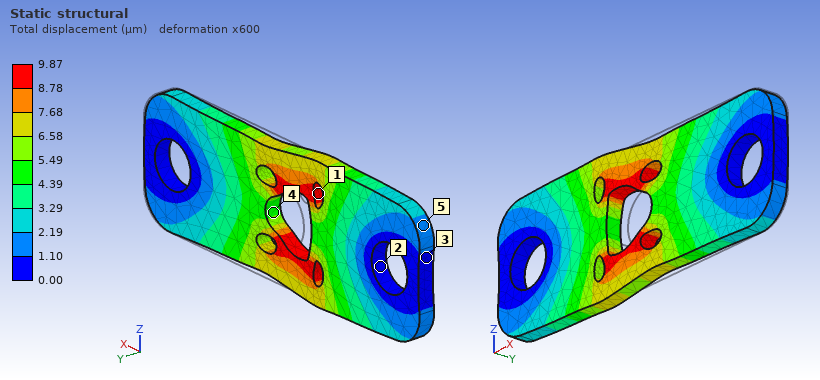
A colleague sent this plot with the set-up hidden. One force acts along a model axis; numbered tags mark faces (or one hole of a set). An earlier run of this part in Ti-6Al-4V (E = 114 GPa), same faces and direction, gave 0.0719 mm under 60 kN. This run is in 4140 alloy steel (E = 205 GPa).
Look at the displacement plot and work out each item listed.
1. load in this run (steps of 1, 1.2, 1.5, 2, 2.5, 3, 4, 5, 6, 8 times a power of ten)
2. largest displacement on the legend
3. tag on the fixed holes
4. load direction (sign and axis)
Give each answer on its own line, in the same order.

15 kN
9.87 µm
2
-X
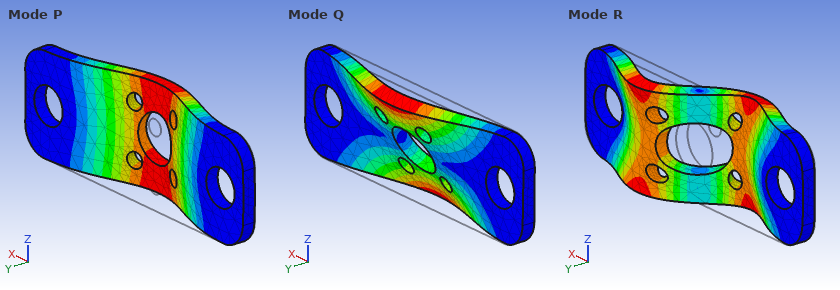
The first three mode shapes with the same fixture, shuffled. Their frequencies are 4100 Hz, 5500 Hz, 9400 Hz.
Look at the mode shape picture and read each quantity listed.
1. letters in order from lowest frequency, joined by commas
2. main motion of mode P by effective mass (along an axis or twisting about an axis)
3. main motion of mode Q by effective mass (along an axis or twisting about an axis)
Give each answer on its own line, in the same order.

P, Q, R
along Y
twisting about X
